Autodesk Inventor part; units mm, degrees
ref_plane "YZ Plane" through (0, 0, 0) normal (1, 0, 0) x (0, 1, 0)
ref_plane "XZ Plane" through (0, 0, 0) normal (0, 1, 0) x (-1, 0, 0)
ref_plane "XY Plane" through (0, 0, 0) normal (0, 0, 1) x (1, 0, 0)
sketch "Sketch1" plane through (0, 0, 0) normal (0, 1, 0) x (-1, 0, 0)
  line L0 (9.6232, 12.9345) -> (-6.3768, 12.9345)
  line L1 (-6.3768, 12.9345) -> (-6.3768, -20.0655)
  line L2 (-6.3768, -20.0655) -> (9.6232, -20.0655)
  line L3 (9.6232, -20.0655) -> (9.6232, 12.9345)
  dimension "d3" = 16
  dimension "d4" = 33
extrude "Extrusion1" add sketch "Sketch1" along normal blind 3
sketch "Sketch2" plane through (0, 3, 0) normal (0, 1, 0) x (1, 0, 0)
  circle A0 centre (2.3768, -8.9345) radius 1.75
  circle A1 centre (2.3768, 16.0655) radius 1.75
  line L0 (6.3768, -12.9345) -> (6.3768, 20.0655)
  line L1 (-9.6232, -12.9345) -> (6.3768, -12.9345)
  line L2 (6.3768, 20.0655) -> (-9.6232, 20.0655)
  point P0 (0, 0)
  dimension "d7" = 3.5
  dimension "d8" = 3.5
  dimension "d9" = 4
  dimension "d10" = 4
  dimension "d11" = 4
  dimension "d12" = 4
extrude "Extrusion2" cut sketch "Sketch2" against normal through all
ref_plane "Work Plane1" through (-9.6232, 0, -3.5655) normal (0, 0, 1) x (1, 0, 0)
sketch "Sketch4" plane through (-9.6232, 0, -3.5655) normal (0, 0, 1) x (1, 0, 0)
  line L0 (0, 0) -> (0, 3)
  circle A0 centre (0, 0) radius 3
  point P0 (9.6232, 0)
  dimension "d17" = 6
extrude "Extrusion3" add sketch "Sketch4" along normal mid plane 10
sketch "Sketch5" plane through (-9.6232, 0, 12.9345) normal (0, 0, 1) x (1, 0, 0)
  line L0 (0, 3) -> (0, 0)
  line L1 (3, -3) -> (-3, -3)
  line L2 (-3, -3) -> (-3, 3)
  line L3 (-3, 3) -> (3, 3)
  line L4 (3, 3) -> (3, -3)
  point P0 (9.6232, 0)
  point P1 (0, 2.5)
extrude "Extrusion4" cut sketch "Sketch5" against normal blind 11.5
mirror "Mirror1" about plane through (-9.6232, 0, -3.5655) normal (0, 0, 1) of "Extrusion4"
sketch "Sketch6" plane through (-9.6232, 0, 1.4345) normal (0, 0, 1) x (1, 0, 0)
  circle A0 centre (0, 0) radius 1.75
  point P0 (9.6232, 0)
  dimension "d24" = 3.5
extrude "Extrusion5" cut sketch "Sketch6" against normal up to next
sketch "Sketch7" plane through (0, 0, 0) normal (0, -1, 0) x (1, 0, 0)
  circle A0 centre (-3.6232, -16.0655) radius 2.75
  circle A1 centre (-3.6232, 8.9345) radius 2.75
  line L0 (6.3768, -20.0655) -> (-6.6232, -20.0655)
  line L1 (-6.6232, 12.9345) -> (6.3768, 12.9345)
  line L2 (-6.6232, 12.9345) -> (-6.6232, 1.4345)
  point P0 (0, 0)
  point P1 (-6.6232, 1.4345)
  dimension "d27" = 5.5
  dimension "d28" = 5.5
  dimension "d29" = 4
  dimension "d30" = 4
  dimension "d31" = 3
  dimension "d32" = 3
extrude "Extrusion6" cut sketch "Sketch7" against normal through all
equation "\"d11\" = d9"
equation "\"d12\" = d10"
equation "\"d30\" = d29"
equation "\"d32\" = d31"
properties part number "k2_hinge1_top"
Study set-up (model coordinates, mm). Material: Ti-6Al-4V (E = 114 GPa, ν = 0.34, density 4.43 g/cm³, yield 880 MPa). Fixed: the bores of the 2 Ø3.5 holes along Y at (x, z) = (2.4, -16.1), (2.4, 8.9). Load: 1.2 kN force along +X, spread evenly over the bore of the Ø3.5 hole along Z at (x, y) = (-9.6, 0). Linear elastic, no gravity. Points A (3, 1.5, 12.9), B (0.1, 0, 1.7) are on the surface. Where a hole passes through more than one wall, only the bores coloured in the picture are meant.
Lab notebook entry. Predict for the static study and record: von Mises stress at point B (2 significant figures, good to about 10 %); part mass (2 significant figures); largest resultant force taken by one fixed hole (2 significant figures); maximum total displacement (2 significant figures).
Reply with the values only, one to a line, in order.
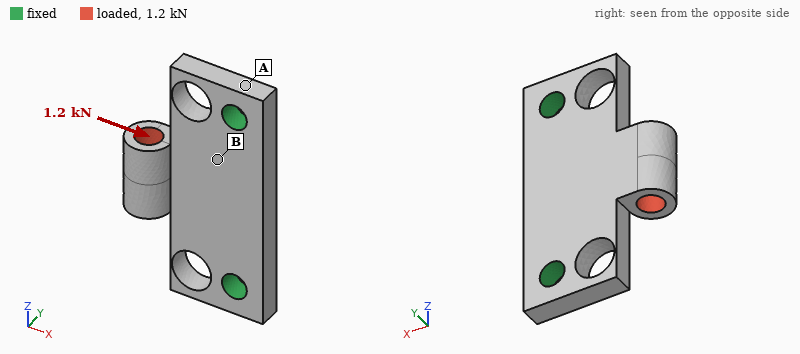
72 MPa
5.7 g
680 N
70 µm
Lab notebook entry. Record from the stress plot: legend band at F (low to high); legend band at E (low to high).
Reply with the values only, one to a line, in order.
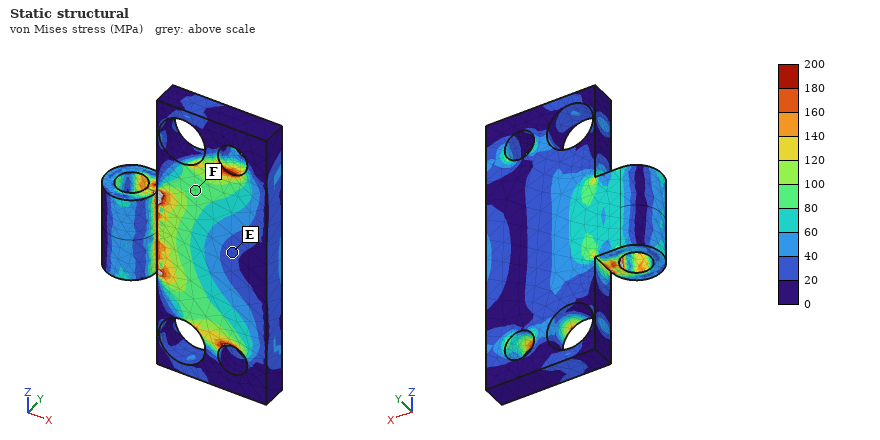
80 to 100 MPa
20 to 40 MPa
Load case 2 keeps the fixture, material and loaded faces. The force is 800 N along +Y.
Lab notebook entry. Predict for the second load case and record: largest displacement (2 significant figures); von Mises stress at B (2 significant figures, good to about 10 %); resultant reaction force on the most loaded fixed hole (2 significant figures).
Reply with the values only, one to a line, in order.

0.24 mm
200 MPa
400 N
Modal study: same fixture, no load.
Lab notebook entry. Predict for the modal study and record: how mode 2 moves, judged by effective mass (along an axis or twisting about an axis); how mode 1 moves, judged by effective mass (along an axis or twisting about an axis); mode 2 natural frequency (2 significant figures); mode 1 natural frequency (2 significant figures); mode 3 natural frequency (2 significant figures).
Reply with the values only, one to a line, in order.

along Y
along Y
27 kHz
9700 Hz
31 kHz
